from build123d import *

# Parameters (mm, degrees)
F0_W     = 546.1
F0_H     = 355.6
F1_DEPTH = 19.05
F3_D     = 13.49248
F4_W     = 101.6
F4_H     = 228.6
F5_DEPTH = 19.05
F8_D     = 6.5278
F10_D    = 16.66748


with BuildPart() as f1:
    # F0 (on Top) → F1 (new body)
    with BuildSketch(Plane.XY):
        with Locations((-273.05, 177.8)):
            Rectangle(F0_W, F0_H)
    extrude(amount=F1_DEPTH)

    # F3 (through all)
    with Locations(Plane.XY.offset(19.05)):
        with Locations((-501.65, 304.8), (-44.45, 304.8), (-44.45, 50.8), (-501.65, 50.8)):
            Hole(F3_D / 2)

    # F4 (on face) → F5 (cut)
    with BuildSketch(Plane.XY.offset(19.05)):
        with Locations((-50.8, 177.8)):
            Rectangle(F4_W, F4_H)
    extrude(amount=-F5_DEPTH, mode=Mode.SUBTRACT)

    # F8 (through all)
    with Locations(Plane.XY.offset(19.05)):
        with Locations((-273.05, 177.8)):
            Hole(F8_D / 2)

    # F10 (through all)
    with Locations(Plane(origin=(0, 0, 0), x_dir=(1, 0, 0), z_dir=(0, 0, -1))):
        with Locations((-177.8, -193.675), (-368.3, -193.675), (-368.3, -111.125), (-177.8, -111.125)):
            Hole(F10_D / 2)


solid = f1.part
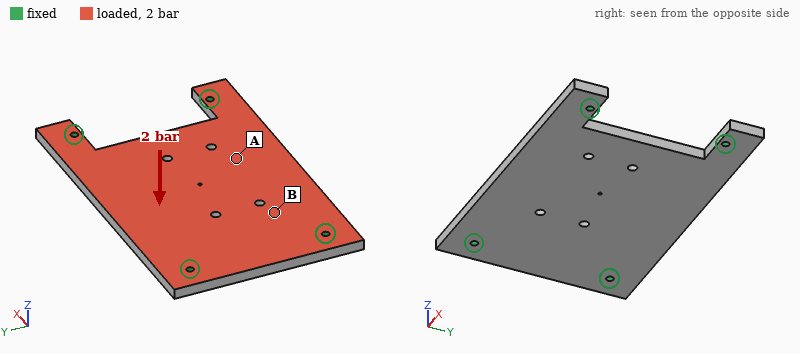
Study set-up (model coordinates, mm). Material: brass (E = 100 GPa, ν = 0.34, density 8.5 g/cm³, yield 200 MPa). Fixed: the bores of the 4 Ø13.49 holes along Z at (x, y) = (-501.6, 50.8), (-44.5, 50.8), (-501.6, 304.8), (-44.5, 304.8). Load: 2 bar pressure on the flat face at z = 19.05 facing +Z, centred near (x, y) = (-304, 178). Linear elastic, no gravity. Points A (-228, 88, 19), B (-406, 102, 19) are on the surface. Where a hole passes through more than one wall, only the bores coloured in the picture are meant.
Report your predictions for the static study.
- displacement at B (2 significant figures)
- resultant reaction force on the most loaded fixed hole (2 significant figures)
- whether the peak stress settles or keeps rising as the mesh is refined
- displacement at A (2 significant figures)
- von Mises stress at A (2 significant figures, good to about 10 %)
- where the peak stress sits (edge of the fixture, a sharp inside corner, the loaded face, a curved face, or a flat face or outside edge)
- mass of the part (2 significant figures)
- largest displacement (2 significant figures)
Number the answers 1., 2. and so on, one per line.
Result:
1. 0.33 mm
2. 9.9 kN
3. keeps rising
4. 0.60 mm
5. 31 MPa
6. edge of the fixture
7. 27 kg
8. 0.64 mm
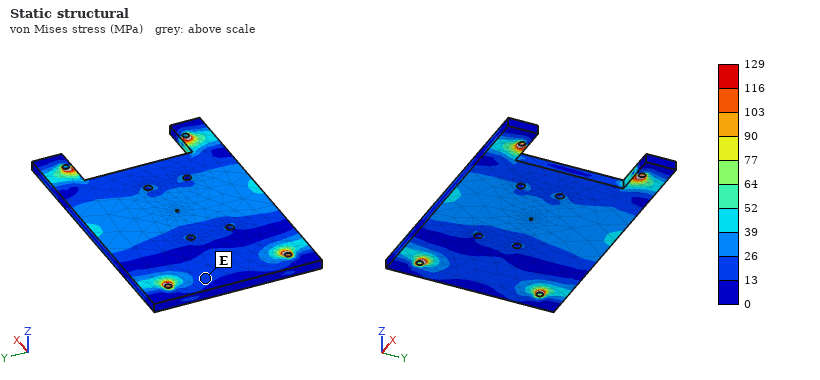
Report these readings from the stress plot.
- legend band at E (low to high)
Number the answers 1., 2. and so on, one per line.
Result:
1. 13 to 26 MPa
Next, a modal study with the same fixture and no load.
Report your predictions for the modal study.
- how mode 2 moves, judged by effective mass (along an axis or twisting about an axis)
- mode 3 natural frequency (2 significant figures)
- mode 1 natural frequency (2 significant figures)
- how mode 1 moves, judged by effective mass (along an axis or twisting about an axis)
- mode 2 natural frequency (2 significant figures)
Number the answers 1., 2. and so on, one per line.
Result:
1. twisting about X
2. 610 Hz
3. 250 Hz
4. along Z
5. 370 Hz
